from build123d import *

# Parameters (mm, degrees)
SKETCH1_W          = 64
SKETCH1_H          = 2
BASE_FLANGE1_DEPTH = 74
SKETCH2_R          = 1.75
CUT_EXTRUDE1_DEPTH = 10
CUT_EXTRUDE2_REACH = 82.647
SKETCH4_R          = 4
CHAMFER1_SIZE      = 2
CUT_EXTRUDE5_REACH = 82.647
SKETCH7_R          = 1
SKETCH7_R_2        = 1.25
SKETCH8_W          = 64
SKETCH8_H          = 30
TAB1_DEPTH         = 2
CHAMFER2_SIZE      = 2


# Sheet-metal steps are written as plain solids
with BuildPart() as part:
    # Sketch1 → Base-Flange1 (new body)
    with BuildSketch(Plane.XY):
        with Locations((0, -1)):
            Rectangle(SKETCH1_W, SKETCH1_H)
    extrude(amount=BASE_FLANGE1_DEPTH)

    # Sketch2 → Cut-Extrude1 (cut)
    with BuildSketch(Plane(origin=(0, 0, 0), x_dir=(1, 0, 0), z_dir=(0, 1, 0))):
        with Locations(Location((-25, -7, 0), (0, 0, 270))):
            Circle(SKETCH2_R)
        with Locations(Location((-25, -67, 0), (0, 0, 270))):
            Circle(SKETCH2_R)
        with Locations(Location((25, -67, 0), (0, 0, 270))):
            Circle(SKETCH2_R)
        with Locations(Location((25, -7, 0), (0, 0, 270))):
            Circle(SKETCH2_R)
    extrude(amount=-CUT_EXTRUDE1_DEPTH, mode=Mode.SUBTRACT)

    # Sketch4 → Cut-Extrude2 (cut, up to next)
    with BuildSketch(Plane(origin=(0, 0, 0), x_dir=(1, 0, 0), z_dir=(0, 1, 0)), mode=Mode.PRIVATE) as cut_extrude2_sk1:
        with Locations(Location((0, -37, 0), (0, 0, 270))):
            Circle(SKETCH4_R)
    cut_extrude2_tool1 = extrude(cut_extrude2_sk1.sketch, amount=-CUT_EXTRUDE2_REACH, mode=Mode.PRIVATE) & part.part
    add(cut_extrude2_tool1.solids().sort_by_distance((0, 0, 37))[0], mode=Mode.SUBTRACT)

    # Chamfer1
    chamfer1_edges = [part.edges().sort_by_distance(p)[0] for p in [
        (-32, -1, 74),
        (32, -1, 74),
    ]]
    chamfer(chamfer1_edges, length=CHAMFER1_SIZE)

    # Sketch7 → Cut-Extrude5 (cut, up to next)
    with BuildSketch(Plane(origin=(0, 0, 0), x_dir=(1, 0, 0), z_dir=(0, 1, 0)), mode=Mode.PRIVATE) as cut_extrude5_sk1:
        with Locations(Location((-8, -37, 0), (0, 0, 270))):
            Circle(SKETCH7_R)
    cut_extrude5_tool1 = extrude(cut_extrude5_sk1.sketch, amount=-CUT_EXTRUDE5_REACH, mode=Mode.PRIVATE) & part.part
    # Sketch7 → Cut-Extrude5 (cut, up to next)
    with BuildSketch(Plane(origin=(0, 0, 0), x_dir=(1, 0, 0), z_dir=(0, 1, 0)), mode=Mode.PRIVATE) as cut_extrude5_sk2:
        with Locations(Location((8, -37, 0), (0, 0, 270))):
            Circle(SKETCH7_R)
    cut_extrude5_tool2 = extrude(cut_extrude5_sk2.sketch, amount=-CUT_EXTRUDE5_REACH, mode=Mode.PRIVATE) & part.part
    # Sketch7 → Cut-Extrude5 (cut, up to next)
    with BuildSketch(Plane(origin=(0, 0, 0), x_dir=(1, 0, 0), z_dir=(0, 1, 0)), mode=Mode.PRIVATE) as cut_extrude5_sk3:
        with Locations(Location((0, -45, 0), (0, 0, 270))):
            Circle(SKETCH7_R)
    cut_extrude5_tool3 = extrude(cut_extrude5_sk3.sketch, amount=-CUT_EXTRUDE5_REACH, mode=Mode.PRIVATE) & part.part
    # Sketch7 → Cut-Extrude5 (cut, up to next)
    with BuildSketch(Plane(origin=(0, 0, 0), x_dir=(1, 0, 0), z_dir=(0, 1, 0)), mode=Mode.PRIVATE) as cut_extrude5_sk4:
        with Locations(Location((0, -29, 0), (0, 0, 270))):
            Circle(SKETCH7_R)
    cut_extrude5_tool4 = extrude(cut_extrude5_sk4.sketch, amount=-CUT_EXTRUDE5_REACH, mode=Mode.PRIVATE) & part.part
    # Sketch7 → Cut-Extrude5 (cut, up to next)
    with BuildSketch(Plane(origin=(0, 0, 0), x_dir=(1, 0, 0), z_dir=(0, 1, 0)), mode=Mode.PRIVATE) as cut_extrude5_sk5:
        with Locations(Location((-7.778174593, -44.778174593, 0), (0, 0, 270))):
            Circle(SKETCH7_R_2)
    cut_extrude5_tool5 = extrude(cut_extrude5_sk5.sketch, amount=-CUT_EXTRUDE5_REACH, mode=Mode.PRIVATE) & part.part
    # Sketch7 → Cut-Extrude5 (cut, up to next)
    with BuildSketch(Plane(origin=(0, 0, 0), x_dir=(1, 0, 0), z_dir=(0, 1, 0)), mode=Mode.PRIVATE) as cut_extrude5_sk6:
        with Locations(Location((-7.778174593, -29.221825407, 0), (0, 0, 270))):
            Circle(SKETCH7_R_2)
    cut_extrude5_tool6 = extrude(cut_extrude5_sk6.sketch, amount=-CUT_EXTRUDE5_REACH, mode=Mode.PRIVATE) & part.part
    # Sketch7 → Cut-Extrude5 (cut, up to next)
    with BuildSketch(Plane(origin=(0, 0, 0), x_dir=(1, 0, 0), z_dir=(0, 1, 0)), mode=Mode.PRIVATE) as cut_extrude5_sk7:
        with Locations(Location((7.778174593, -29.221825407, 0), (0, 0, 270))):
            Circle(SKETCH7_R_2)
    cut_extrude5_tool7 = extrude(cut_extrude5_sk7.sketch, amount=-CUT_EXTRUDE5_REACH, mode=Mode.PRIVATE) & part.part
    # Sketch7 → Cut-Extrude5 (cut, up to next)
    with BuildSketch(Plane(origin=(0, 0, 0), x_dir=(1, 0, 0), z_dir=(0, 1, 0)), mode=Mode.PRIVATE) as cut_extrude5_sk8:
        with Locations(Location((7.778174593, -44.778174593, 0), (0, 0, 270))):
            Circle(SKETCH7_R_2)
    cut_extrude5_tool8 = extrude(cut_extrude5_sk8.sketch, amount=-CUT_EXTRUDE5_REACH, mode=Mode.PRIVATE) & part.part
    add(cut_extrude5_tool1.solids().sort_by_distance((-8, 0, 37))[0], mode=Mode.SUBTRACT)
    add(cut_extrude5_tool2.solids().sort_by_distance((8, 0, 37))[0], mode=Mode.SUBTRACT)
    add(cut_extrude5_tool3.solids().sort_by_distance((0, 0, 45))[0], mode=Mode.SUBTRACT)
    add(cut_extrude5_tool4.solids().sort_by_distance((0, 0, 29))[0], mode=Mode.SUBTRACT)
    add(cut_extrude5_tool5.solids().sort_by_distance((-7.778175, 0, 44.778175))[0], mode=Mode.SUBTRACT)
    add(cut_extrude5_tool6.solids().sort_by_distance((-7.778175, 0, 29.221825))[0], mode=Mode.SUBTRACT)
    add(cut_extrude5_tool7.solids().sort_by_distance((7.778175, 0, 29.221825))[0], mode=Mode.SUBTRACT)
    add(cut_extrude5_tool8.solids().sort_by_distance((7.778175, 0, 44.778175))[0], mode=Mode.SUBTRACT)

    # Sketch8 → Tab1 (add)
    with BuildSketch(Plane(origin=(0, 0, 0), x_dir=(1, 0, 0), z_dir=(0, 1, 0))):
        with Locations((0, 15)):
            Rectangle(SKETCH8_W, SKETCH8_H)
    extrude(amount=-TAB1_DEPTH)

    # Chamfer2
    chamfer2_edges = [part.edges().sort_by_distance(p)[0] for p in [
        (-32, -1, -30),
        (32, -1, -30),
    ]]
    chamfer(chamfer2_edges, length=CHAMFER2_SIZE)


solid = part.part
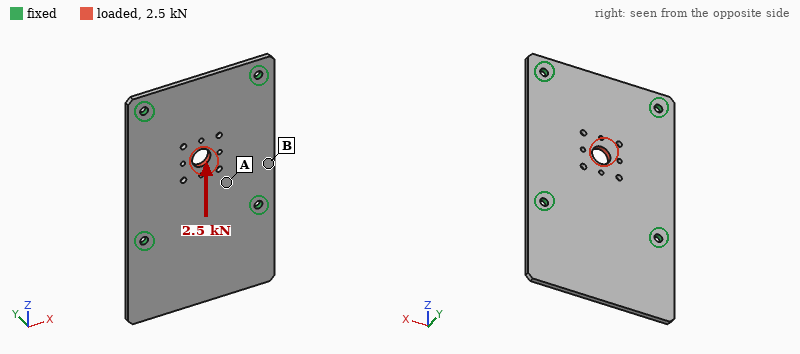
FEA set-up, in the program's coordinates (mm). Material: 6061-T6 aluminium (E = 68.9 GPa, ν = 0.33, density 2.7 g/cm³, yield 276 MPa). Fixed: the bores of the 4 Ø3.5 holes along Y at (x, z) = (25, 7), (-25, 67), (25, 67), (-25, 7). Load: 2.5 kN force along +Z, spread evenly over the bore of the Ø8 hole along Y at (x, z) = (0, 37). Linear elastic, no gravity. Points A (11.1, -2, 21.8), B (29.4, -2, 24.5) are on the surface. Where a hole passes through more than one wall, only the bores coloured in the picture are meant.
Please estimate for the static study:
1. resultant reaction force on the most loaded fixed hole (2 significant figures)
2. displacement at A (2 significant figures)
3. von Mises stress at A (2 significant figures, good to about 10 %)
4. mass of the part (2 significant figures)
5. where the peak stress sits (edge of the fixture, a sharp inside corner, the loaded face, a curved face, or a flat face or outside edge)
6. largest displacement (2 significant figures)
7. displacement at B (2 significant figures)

710 N
6.5 µm
18 MPa
35 g
a curved face
16 µm
3.2 µm
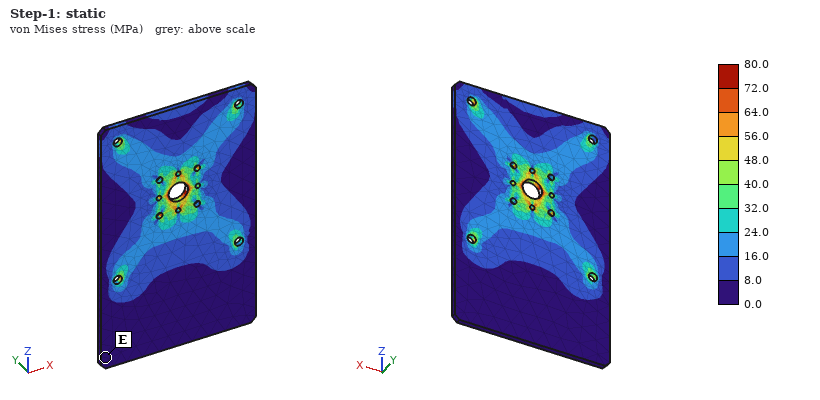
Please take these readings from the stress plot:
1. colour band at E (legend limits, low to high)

0.0 to 8.0 MPa
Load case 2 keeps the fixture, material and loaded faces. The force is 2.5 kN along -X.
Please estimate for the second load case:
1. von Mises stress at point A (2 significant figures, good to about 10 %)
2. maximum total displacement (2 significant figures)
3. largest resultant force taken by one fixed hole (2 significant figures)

23 MPa
20 µm
730 N
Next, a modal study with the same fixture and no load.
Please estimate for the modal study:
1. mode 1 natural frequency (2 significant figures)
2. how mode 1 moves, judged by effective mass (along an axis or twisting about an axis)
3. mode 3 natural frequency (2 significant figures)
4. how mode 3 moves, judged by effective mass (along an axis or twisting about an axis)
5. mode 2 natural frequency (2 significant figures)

1100 Hz
along Y
2300 Hz
along Y
2100 Hz
